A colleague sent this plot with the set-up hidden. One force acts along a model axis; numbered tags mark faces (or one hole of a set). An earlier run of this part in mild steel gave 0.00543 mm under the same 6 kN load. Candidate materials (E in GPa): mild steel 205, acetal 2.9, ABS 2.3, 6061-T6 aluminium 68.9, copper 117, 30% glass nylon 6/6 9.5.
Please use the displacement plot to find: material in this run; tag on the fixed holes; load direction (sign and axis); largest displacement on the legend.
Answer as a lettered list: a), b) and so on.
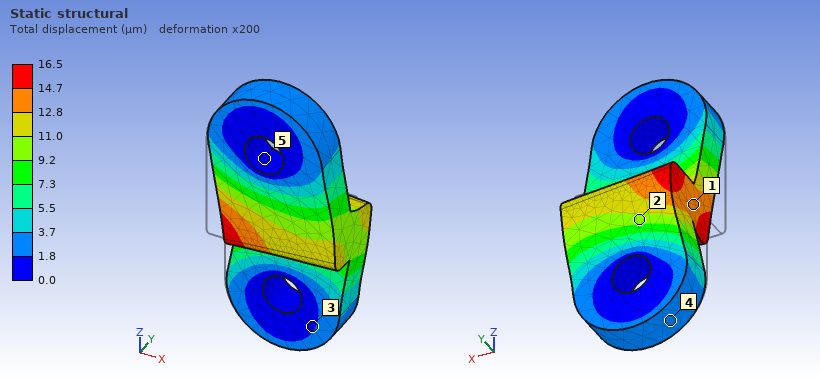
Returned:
a) 6061-T6 aluminium
b) 5
c) +X
d) 16.5 µm
